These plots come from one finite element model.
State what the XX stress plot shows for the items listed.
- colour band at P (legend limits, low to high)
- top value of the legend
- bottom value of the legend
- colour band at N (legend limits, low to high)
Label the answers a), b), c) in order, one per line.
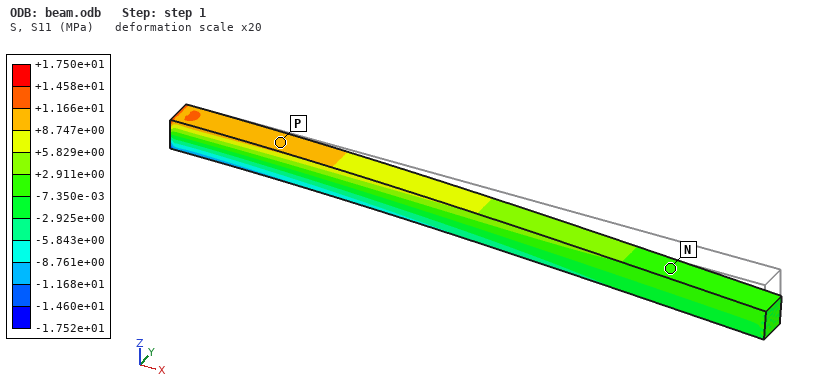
a) +8.747e+00 to +1.166e+01 MPa
b) +1.750e+01 MPa
c) -1.752e+01 MPa
d) -7.350e-03 to +2.911e+00 MPa
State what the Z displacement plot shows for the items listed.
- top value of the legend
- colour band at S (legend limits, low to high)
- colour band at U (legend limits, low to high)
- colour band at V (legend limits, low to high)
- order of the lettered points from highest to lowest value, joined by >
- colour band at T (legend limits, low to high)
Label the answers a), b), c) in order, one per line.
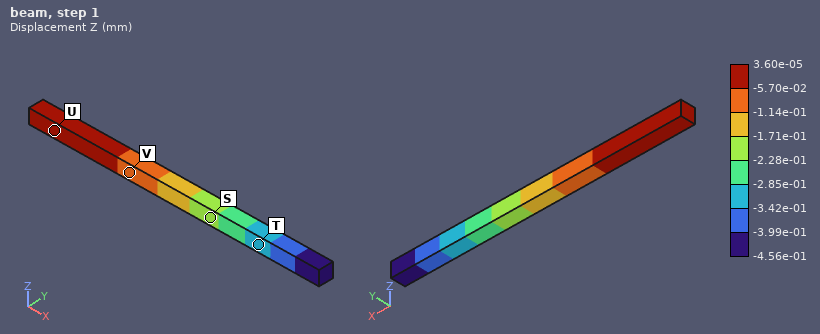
a) 3.60e-05 mm
b) -2.28e-01 to -1.71e-01 mm
c) -5.70e-02 to 3.60e-05 mm
d) -1.14e-01 to -5.70e-02 mm
e) U > V > S > T
f) -3.42e-01 to -2.85e-01 mm
